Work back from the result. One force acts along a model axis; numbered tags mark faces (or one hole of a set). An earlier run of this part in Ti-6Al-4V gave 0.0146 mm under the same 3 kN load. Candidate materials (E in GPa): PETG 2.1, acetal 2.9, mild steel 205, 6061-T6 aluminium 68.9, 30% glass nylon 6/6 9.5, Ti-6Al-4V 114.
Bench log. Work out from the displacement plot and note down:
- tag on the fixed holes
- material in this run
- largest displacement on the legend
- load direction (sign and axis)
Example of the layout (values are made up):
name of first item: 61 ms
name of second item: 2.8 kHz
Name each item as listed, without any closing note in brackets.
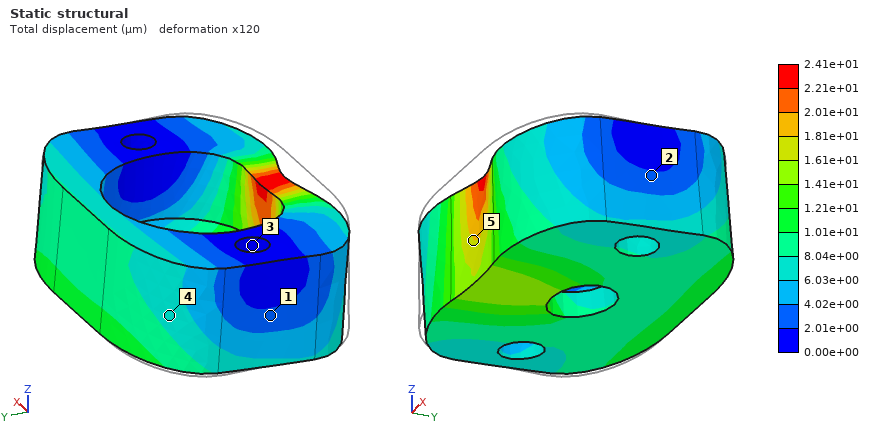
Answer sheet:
tag on the fixed holes: 3
material in this run: 6061-T6 aluminium
largest displacement on the legend: 2.41e+01 µm
load direction: +Y
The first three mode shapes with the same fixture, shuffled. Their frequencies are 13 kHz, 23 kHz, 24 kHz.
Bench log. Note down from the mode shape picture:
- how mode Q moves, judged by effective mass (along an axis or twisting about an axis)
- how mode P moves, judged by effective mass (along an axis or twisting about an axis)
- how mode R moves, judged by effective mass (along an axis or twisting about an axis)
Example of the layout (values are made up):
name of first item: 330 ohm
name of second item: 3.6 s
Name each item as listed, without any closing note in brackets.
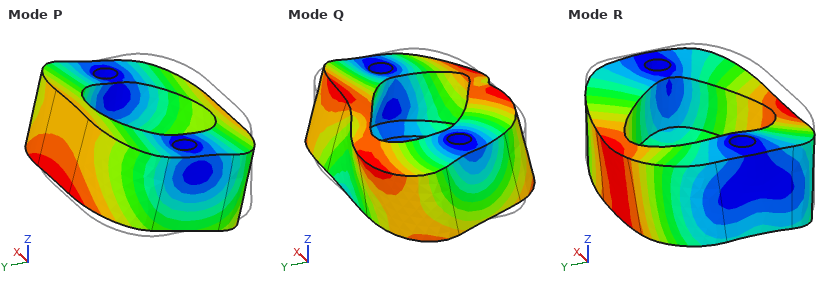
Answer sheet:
how mode Q moves, judged by effective mass: twisting about Z
how mode P moves, judged by effective mass: along Y
how mode R moves, judged by effective mass: along Z
